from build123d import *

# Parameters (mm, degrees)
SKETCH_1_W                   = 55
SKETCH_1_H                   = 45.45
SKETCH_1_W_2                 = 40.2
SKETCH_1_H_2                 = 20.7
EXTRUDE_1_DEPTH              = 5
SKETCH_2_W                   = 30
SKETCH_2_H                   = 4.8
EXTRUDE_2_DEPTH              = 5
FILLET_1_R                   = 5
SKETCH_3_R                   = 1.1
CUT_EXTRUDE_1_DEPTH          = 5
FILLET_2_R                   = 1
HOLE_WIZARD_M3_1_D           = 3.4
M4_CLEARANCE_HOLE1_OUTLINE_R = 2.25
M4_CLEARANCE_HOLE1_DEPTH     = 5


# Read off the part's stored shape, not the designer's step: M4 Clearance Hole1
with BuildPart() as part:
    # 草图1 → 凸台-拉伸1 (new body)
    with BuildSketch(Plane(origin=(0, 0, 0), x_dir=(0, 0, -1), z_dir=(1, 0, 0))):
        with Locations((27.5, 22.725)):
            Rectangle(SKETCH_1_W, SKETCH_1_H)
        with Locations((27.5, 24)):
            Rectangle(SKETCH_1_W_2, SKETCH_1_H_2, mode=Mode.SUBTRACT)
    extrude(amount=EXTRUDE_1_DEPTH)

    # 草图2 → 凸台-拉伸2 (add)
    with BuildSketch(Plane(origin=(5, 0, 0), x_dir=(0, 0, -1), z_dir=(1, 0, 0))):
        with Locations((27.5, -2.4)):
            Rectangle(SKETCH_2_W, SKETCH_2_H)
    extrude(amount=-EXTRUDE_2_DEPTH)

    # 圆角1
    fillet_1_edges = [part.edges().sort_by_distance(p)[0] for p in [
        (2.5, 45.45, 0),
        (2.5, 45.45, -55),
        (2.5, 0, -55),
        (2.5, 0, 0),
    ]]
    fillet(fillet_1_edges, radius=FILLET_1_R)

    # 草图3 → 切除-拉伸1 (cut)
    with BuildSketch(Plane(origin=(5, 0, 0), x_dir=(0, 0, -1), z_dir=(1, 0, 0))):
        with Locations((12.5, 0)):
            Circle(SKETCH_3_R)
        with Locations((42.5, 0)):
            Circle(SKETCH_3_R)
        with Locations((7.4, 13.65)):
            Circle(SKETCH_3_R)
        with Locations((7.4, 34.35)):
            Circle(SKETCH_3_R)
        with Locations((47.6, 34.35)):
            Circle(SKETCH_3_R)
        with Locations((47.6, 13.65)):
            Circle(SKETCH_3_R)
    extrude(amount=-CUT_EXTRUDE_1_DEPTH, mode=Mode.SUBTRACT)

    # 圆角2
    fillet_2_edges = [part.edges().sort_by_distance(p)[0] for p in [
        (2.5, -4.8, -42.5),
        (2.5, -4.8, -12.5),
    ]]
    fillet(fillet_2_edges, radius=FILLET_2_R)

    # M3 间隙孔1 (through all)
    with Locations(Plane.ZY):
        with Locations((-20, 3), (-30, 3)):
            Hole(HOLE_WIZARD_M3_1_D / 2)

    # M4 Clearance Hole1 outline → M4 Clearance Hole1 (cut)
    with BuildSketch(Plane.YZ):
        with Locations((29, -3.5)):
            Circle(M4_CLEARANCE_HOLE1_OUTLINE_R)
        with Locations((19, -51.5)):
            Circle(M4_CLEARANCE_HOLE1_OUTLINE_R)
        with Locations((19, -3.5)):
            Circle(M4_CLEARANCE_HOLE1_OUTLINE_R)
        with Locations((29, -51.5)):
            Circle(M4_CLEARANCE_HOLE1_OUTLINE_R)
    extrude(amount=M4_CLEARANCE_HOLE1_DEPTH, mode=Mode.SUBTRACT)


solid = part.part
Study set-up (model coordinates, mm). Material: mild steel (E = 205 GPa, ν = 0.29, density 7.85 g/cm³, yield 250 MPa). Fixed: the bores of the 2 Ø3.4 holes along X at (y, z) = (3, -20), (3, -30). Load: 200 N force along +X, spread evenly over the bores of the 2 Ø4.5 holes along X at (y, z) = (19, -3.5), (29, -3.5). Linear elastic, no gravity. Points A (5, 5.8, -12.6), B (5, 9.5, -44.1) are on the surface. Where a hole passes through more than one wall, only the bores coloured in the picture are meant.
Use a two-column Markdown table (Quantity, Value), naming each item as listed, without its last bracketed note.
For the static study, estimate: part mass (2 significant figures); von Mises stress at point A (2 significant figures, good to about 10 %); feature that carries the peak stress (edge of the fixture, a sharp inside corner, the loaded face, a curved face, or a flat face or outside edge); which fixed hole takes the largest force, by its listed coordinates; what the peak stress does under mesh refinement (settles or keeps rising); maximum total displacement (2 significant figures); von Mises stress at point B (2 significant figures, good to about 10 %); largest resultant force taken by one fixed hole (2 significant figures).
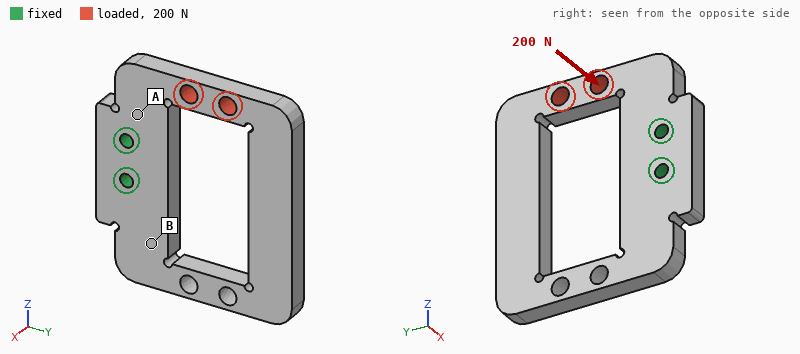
| Quantity | Value |
|---|---|
| part mass | 66 g |
| von Mises stress at point A | 63 MPa |
| feature that carries the peak stress | edge of the fixture |
| which fixed hole takes the largest force, by its listed coordinates | (3, -20) |
| what the peak stress does under mesh refinement | keeps rising |
| maximum total displacement | 0.11 mm |
| von Mises stress at point B | 12 MPa |
| largest resultant force taken by one fixed hole | 300 N |
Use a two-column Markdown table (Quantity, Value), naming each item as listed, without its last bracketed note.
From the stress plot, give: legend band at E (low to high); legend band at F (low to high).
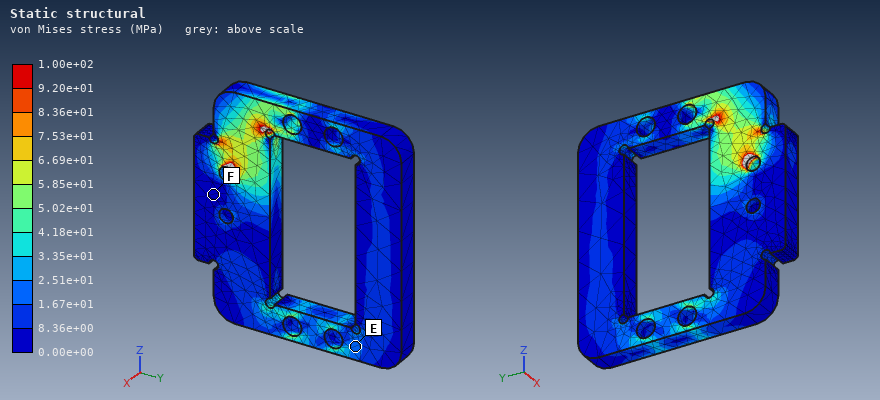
| Quantity | Value |
|---|---|
| legend band at E | 1.67e+01 to 2.51e+01 MPa |
| legend band at F | 0.00e+00 to 8.36e+00 MPa |
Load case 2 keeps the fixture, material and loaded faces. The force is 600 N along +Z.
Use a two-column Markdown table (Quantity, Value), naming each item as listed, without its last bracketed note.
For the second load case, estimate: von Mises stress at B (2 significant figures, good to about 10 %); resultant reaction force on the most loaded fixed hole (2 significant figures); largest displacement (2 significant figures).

| Quantity | Value |
|---|---|
| von Mises stress at B | 12 MPa |
| resultant reaction force on the most loaded fixed hole | 940 N |
| largest displacement | 37 µm |
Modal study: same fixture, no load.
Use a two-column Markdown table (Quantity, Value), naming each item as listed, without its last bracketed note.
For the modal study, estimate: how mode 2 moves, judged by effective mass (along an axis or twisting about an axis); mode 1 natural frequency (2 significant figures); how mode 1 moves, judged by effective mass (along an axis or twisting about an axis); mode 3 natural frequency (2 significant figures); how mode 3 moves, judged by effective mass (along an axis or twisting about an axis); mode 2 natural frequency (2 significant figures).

| Quantity | Value |
|---|---|
| how mode 2 moves, judged by effective mass | twisting about Y |
| mode 1 natural frequency | 1100 Hz |
| how mode 1 moves, judged by effective mass | along X |
| mode 3 natural frequency | 2900 Hz |
| how mode 3 moves, judged by effective mass | along Z |
| mode 2 natural frequency | 2500 Hz |
